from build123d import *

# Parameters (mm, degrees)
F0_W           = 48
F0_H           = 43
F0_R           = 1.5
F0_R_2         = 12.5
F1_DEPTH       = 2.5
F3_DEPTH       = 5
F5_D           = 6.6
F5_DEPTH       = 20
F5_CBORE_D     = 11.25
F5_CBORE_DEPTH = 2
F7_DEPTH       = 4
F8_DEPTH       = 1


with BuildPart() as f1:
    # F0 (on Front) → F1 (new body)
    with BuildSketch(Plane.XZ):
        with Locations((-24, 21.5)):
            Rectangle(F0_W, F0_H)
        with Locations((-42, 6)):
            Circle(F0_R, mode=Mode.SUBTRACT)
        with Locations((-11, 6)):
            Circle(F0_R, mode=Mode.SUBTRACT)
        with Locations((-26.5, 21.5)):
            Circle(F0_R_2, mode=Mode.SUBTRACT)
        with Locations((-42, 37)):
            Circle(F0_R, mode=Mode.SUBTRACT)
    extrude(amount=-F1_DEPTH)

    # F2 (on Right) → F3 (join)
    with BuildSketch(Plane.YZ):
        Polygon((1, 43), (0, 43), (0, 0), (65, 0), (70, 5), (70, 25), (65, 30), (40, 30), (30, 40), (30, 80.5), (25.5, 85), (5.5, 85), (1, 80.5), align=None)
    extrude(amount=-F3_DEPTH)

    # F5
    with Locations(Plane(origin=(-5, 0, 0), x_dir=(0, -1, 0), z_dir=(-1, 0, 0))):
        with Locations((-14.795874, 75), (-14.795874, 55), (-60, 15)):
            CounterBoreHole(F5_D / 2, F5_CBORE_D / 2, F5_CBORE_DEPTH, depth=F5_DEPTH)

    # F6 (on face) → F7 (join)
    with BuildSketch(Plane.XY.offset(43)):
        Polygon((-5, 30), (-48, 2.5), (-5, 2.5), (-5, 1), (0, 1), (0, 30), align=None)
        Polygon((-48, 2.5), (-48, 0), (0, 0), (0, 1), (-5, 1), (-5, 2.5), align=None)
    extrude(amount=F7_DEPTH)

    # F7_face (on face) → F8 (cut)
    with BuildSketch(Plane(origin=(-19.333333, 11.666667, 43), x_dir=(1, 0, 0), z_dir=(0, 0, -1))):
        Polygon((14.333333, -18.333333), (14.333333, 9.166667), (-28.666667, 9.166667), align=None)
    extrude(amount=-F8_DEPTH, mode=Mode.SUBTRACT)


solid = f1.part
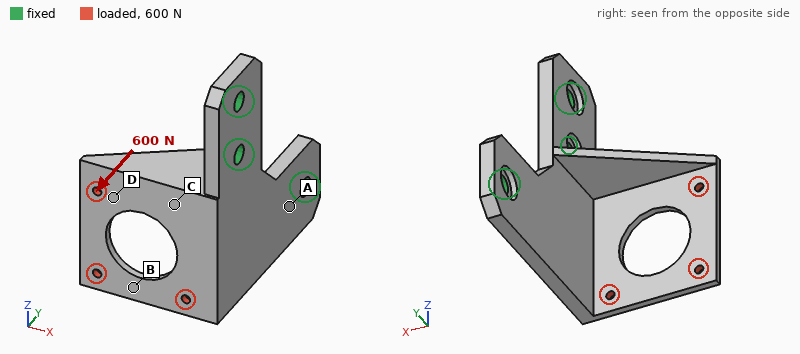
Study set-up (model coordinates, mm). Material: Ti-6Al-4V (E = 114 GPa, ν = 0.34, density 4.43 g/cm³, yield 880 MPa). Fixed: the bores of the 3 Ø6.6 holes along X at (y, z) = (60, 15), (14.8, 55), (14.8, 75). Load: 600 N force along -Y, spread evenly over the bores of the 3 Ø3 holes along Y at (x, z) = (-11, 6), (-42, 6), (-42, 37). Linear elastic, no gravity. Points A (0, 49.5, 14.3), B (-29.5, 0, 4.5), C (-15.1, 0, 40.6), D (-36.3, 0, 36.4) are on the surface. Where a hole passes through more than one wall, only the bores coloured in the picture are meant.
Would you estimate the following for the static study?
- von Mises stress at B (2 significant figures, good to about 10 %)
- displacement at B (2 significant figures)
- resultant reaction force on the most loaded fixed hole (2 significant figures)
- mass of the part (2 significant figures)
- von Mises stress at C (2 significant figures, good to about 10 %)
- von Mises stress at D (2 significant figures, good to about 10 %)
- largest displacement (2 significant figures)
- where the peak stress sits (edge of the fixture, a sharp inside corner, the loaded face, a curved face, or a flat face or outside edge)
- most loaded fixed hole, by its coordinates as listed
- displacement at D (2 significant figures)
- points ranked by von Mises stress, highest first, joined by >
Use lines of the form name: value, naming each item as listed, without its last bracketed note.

von Mises stress at B: 100 MPa
displacement at B: 0.57 mm
resultant reaction force on the most loaded fixed hole: 610 N
mass of the part: 100 g
von Mises stress at C: 56 MPa
von Mises stress at D: 150 MPa
largest displacement: 1.2 mm
where the peak stress sits: the loaded face
most loaded fixed hole, by its coordinates as listed: (60, 15)
displacement at D: 0.22 mm
points ranked by von Mises stress, highest first, joined by >: D > B > C > A
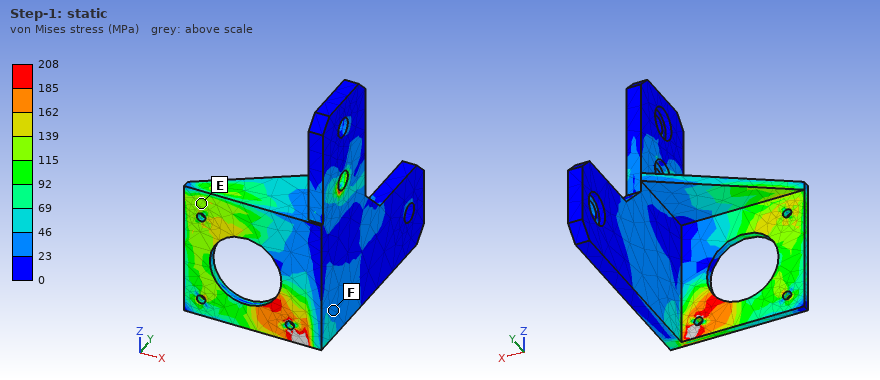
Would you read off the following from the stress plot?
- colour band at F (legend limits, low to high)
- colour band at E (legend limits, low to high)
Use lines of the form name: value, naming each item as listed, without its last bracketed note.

colour band at F: 23 to 46 MPa
colour band at E: 115 to 139 MPa
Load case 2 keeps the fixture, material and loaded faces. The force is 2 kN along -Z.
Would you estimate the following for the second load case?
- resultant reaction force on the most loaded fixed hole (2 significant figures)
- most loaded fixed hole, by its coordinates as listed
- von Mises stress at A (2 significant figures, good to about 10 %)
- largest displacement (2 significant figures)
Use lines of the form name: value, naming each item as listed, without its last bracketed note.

resultant reaction force on the most loaded fixed hole: 1.8 kN
most loaded fixed hole, by its coordinates as listed: (14.8, 75)
von Mises stress at A: 140 MPa
largest displacement: 1.3 mm
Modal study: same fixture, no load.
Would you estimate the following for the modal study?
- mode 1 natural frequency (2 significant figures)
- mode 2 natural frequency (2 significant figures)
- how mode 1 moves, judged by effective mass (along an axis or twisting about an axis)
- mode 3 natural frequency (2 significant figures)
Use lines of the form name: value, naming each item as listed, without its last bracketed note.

mode 1 natural frequency: 1200 Hz
mode 2 natural frequency: 1600 Hz
how mode 1 moves, judged by effective mass: along X
mode 3 natural frequency: 3700 Hz
